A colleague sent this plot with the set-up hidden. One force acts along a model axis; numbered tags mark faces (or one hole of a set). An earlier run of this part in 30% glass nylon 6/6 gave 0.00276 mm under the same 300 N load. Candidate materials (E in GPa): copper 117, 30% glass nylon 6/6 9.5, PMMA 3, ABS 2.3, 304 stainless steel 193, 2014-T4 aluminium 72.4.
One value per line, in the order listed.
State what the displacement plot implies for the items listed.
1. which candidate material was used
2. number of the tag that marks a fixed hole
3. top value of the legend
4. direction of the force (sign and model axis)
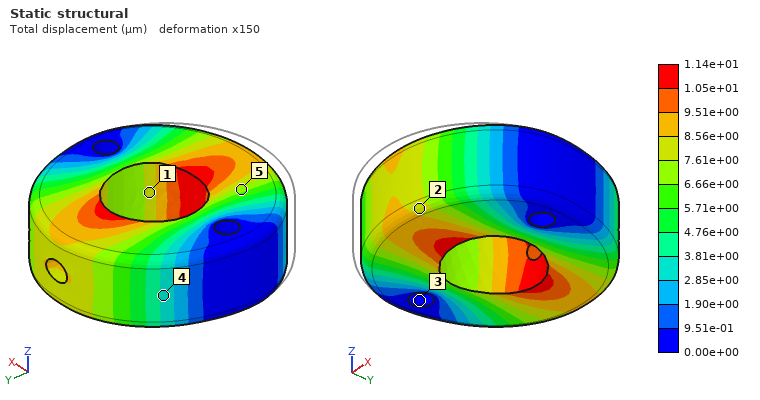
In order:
ABS
3
1.14e+01 µm
+Y
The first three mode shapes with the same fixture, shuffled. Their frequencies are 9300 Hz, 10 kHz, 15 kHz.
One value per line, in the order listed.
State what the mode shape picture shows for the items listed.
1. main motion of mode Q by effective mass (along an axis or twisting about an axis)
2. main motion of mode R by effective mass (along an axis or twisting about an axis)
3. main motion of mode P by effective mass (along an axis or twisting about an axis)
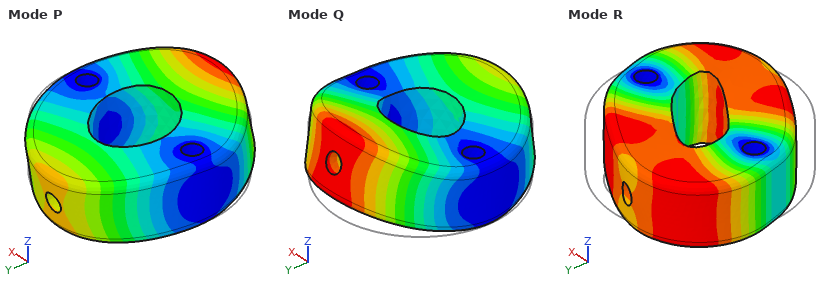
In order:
along Z
twisting about Z
twisting about X
